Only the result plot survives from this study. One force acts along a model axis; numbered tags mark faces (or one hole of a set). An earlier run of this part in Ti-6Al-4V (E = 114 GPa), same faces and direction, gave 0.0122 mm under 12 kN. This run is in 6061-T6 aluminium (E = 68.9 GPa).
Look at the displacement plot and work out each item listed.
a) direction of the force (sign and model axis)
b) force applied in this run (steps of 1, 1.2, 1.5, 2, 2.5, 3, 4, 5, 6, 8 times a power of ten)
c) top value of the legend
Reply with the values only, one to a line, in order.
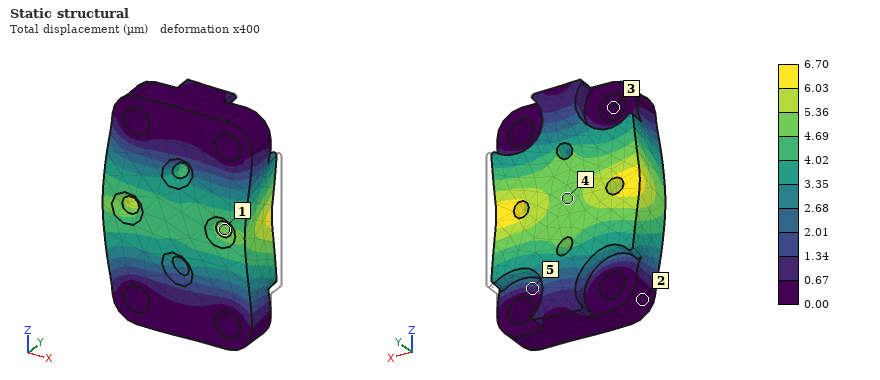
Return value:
-X
4 kN
6.70 µm
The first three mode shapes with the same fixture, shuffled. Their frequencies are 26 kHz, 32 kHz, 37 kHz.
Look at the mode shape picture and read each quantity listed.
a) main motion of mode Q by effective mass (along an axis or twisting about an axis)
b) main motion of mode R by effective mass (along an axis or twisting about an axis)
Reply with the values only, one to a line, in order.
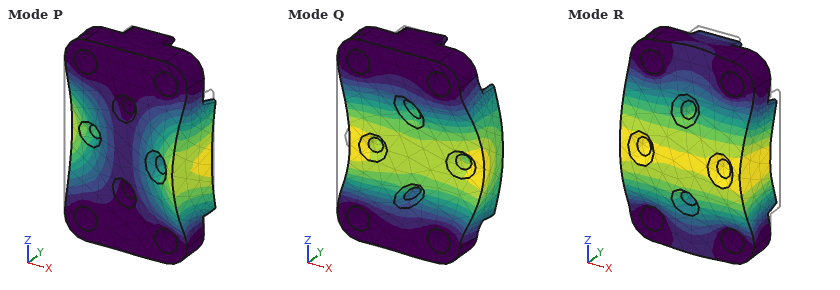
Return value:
along X
along Y
